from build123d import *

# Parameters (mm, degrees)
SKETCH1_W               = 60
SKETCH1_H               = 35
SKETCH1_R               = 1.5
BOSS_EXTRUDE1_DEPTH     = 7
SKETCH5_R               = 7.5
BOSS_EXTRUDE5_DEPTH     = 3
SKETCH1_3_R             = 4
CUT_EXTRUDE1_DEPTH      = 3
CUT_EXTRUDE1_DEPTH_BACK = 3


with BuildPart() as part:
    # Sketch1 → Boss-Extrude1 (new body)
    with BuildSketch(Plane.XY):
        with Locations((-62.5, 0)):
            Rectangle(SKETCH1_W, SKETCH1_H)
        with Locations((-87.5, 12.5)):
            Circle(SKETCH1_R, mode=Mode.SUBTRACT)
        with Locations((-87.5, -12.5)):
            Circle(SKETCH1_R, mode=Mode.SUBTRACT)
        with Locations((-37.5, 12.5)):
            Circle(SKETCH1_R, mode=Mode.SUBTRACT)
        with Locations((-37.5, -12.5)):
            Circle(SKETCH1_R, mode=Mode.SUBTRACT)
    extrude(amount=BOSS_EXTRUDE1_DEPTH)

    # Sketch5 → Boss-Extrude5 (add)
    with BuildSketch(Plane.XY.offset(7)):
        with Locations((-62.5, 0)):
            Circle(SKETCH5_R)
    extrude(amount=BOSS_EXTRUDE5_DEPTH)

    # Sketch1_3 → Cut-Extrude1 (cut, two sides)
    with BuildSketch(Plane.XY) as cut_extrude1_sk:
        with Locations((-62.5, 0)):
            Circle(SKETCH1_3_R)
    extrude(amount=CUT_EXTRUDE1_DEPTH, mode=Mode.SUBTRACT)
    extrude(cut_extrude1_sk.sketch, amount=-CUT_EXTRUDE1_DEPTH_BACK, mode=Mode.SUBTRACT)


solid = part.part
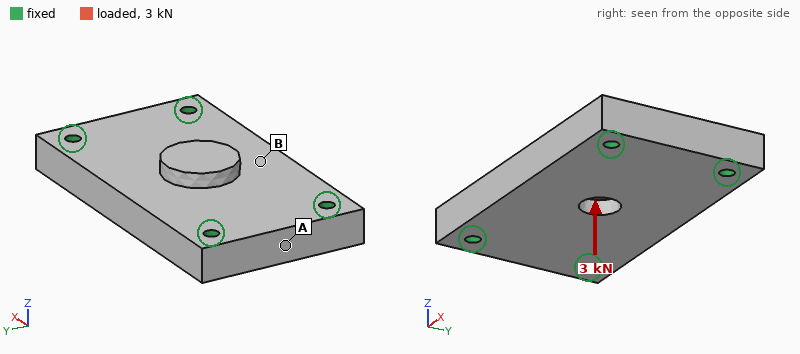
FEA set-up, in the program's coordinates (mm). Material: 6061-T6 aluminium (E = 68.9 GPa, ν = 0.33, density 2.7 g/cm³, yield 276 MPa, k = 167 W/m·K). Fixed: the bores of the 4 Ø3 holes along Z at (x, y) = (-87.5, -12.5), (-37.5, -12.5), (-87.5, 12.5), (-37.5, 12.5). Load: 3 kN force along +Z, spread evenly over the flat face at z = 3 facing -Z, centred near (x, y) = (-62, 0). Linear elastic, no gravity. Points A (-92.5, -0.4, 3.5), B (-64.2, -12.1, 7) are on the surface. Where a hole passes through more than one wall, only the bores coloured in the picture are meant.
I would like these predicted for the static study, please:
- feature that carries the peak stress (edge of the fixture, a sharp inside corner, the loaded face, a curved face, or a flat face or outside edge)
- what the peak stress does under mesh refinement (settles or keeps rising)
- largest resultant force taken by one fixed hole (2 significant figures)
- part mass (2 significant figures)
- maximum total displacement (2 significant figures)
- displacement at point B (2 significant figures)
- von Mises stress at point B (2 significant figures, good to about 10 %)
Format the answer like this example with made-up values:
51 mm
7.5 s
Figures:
edge of the fixture
keeps rising
770 N
40 g
44 µm
34 µm
42 MPa
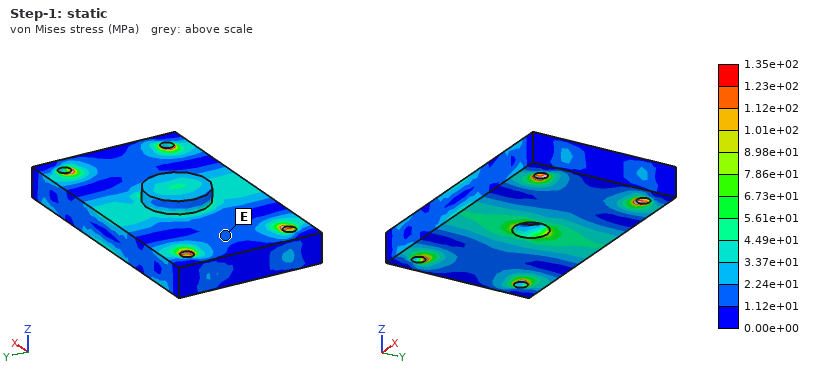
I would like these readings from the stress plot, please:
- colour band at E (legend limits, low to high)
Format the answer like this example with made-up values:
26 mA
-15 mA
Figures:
1.12e+01 to 2.24e+01 MPa
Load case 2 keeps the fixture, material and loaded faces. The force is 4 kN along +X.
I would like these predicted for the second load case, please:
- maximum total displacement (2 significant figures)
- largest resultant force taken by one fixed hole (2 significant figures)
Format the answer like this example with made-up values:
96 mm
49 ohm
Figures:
12 µm
1.0 kN
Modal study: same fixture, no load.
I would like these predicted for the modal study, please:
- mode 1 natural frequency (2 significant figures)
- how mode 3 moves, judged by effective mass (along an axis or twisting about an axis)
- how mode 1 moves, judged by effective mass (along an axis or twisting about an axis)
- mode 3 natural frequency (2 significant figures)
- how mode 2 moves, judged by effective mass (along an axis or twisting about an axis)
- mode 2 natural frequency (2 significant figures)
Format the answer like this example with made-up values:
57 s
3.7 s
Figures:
11 kHz
along Y
along Z
25 kHz
twisting about X
16 kHz
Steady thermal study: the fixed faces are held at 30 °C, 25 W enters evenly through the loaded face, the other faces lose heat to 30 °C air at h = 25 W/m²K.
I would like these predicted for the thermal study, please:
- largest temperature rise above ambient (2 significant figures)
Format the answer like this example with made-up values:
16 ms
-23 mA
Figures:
16 K
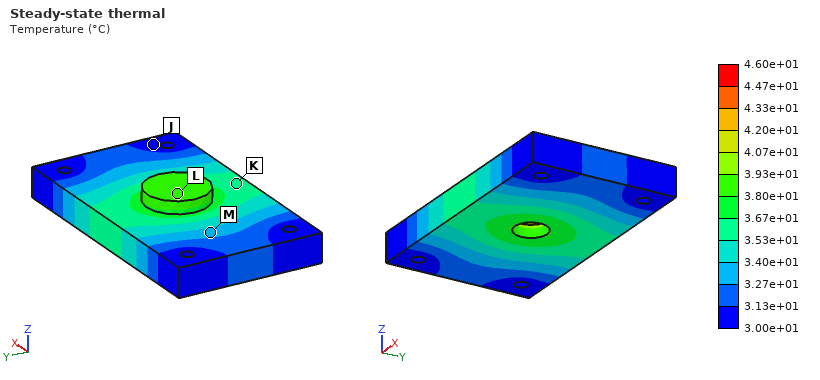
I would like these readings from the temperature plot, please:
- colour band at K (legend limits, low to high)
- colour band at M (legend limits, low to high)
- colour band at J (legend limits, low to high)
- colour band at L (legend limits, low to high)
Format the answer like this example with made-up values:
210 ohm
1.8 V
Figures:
3.53e+01 to 3.67e+01 °C
3.27e+01 to 3.40e+01 °C
3.00e+01 to 3.13e+01 °C
3.80e+01 to 3.93e+01 °C
